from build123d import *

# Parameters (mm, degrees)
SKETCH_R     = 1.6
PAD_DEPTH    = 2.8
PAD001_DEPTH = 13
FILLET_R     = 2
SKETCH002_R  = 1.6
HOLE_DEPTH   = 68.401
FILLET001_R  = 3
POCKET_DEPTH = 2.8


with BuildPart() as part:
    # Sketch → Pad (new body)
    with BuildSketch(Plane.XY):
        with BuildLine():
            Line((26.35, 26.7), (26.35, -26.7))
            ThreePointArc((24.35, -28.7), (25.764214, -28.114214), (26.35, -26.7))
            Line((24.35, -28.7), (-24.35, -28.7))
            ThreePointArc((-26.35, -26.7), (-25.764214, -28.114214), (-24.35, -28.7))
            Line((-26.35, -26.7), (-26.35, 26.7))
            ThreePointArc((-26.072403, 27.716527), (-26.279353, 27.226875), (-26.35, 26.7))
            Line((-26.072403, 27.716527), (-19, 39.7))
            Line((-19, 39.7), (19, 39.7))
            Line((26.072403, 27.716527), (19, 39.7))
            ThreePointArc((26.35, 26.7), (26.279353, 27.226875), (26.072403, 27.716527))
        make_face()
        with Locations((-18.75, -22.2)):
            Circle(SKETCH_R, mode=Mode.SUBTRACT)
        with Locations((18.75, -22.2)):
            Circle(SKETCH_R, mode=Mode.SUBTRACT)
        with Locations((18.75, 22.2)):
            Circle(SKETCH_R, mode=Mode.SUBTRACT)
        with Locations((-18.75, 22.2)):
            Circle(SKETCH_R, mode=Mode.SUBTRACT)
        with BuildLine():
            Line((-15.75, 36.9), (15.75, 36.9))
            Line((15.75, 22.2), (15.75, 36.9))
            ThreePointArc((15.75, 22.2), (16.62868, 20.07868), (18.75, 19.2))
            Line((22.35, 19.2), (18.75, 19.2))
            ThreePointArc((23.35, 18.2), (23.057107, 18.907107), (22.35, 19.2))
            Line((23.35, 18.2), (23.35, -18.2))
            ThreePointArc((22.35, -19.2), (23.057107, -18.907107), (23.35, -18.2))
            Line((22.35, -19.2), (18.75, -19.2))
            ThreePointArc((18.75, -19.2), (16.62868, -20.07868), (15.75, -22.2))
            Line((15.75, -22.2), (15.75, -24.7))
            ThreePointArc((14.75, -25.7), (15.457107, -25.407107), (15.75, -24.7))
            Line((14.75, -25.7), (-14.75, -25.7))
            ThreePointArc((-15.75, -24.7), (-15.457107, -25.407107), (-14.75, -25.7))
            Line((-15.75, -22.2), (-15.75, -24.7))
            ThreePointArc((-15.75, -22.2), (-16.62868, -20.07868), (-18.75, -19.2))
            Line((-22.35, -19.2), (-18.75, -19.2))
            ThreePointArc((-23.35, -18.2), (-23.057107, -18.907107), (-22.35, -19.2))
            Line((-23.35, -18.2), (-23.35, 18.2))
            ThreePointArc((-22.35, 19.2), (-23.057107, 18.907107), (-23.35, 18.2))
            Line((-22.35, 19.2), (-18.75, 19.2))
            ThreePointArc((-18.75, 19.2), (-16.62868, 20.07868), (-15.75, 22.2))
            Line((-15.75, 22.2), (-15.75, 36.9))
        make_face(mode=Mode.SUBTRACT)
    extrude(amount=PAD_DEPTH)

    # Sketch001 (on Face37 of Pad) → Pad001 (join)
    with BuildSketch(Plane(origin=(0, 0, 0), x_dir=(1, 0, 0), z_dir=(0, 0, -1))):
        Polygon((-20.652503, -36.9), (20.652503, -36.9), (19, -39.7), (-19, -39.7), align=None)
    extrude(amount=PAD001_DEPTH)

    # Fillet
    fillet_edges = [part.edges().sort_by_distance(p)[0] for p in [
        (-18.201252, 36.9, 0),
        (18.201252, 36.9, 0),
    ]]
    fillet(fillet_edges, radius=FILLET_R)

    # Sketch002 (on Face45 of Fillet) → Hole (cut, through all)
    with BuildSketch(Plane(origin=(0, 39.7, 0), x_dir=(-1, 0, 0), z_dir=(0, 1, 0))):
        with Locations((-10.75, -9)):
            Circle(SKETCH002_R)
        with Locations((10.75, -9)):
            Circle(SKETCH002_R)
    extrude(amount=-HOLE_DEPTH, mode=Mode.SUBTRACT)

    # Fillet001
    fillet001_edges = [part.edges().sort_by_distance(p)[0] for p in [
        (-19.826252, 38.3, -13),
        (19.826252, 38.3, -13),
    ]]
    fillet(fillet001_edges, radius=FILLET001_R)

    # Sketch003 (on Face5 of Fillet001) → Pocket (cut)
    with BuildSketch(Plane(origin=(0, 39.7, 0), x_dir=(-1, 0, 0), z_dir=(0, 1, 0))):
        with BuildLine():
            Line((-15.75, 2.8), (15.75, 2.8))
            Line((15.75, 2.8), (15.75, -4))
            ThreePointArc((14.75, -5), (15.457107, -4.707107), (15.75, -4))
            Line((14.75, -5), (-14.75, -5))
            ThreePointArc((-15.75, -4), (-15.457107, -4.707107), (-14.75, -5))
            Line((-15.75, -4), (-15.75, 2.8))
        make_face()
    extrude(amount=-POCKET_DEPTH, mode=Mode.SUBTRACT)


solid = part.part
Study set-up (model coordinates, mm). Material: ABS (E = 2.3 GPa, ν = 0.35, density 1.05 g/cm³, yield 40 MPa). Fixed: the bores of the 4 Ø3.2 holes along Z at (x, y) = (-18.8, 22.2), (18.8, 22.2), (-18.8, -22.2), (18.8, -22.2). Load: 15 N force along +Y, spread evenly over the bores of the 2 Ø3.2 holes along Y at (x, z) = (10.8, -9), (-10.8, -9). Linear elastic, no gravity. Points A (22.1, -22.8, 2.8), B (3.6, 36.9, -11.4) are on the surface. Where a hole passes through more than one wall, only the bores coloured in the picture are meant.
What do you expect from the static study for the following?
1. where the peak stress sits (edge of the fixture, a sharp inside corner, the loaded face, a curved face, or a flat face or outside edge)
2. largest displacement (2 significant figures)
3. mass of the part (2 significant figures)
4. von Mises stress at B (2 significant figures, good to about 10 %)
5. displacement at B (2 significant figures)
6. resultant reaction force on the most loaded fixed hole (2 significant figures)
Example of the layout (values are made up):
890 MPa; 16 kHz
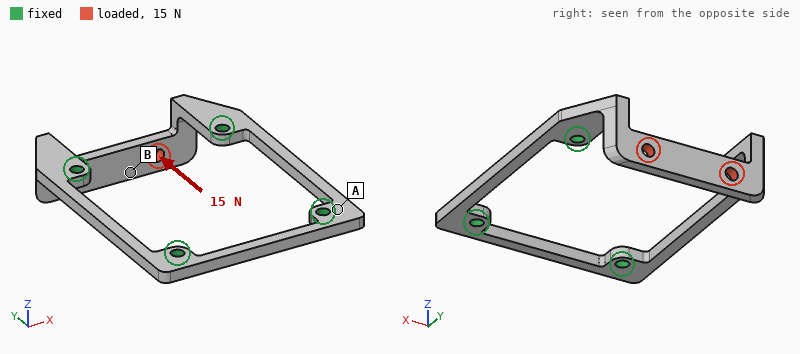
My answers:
a curved face; 0.91 mm; 3.4 g; 2.8 MPa; 0.77 mm; 7.8 N
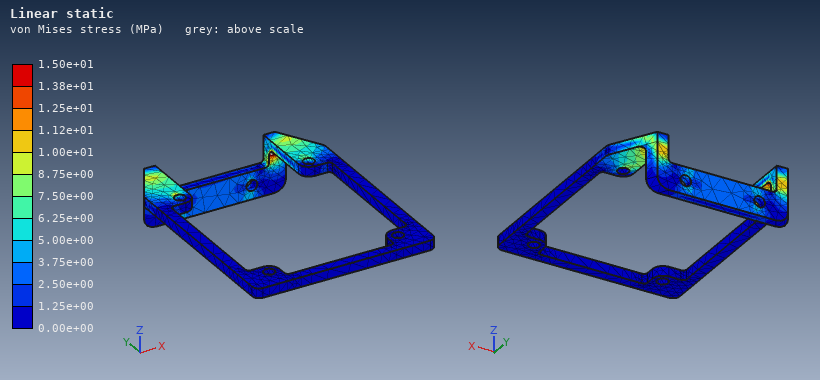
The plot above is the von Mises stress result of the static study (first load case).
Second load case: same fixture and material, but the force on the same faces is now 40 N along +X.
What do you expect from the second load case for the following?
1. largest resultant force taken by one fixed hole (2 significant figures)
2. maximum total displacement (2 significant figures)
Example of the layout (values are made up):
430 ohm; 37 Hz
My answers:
23 N; 0.40 mm
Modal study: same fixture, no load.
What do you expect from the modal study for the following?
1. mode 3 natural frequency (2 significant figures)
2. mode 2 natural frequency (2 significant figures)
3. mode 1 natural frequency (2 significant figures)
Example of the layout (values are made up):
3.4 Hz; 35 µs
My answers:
1800 Hz; 1500 Hz; 730 Hz
